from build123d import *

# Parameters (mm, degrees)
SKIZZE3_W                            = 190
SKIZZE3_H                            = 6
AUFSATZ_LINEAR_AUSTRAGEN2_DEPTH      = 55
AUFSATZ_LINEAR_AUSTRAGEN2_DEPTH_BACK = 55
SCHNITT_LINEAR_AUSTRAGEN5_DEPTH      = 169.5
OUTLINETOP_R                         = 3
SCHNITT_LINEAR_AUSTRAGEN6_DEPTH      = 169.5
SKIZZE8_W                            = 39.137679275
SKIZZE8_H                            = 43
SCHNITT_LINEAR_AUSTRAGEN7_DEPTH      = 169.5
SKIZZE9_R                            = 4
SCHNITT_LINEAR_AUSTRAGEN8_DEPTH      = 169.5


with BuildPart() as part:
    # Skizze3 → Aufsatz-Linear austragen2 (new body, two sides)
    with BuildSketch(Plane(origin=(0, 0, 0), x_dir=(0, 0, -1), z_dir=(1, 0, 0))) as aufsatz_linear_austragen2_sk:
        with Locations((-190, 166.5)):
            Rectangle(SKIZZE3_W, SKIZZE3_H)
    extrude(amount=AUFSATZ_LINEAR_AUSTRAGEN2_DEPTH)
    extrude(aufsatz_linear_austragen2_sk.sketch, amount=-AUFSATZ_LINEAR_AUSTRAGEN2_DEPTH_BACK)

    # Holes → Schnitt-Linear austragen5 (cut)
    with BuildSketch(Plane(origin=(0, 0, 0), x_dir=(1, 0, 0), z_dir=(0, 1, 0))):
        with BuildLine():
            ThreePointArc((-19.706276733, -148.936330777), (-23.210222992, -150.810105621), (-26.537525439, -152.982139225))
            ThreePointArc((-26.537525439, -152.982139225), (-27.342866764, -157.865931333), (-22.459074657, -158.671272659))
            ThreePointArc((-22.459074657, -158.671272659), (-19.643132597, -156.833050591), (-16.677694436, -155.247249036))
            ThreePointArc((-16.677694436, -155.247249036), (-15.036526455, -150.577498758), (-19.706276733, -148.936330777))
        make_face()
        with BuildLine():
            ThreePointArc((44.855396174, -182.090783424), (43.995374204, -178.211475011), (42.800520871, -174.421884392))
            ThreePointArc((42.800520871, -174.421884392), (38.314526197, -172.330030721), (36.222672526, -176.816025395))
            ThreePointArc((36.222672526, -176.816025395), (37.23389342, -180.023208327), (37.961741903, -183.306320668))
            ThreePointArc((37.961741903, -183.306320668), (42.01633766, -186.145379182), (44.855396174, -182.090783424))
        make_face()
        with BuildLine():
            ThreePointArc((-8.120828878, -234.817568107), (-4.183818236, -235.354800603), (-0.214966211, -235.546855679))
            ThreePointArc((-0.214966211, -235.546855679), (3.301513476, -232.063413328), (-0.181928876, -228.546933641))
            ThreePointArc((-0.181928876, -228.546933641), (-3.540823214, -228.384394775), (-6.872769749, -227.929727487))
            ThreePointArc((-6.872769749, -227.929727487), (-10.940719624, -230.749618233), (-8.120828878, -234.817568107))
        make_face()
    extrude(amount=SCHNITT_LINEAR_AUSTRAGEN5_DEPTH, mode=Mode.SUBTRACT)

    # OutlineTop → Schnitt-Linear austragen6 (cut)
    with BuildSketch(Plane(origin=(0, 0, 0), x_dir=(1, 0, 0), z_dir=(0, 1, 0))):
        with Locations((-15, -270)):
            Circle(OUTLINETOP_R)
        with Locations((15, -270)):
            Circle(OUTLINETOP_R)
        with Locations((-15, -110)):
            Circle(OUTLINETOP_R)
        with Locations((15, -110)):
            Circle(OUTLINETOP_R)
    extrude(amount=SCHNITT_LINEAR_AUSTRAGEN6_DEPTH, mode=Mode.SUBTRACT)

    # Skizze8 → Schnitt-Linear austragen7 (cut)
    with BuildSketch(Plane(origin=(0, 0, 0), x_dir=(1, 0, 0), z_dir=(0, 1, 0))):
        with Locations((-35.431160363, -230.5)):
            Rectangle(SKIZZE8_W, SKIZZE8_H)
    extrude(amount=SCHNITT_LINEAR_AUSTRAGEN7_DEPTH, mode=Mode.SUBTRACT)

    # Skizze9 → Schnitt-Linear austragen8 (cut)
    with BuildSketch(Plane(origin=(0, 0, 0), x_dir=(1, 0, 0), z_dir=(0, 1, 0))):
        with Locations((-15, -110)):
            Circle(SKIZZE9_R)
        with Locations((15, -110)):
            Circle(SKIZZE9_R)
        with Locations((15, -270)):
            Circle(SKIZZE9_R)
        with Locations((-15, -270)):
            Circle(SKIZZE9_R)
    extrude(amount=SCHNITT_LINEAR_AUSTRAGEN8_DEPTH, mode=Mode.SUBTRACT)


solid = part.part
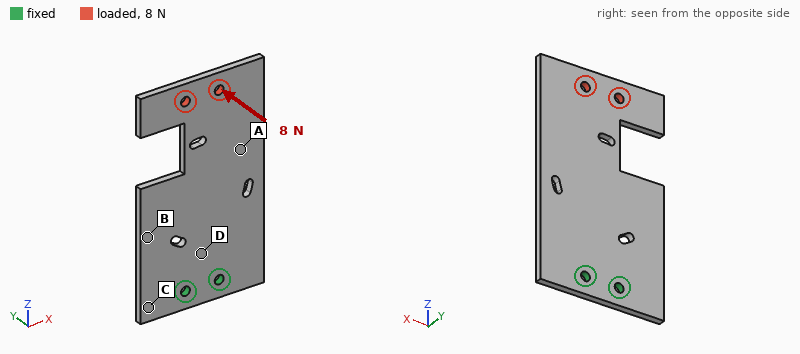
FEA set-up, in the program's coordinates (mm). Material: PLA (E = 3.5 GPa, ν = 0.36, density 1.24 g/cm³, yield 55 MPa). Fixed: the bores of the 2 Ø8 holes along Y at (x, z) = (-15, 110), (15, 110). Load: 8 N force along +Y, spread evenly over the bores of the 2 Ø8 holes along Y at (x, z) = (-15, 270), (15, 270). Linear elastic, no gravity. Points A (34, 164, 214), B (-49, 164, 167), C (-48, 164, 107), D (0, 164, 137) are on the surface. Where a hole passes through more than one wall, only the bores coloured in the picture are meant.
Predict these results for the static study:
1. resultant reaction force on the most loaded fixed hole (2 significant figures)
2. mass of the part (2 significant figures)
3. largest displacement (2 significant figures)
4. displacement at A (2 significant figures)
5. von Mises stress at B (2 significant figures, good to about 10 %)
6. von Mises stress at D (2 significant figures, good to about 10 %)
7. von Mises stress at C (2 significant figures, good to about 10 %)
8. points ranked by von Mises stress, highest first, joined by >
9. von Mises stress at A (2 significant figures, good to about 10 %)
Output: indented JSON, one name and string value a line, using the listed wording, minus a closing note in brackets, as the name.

{
  "resultant reaction force on the most loaded fixed hole": "4.1 N",
  "mass of the part": "140 g",
  "largest displacement": "2.2 mm",
  "displacement at A": "0.86 mm",
  "von Mises stress at B": "1.2 MPa",
  "von Mises stress at D": "1.6 MPa",
  "von Mises stress at C": "0.51 MPa",
  "points ranked by von Mises stress, highest first, joined by >": "D > B > A > C",
  "von Mises stress at A": "0.95 MPa"
}
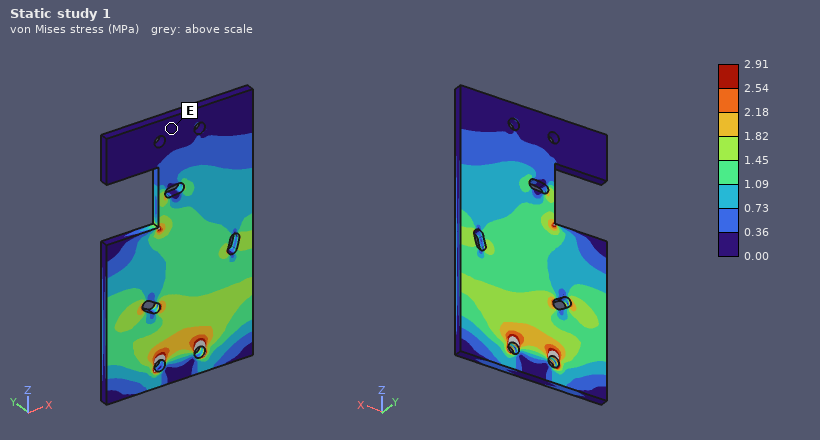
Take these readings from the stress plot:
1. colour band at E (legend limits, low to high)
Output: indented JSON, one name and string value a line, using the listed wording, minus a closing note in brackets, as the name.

{
  "colour band at E": "0.00 to 0.36 MPa"
}
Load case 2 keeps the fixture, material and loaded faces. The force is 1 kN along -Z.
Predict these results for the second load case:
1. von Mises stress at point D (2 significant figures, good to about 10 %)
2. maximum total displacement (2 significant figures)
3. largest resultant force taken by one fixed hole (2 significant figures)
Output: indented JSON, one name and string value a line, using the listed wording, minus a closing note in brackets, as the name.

{
  "von Mises stress at point D": "2.9 MPa",
  "maximum total displacement": "0.42 mm",
  "largest resultant force taken by one fixed hole": "500 N"
}
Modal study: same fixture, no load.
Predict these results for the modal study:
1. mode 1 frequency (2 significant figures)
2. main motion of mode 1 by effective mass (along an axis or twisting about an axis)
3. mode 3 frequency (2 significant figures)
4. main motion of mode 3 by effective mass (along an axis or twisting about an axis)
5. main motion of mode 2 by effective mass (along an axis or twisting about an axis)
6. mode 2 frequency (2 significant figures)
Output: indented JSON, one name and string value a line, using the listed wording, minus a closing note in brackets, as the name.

{
  "mode 1 frequency": "54 Hz",
  "main motion of mode 1 by effective mass": "along Y",
  "mode 3 frequency": "290 Hz",
  "main motion of mode 3 by effective mass": "along Y",
  "main motion of mode 2 by effective mass": "twisting about Z",
  "mode 2 frequency": "170 Hz"
}
